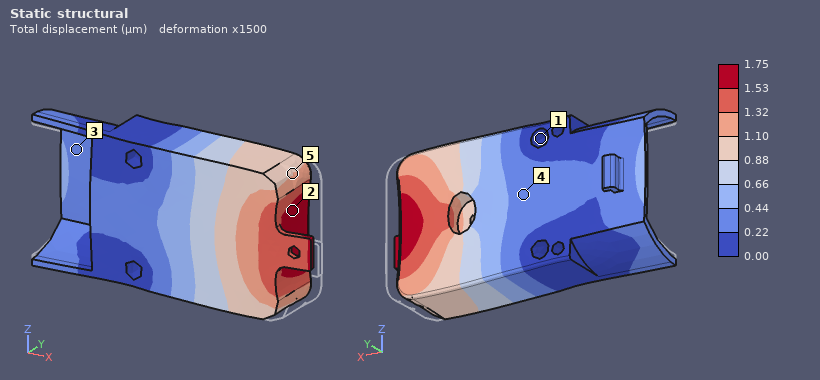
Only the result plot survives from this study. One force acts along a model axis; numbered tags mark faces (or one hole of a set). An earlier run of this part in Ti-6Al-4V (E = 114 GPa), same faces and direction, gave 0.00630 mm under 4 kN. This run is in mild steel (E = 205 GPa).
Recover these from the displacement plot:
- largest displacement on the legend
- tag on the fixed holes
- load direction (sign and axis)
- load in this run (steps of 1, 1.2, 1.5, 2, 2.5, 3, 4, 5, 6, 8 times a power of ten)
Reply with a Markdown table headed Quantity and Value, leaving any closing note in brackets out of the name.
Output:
| Quantity | Value |
|---|---|
| largest displacement on the legend | 1.75 µm |
| tag on the fixed holes | 1 |
| load direction | -X |
| load in this run | 2 kN |
